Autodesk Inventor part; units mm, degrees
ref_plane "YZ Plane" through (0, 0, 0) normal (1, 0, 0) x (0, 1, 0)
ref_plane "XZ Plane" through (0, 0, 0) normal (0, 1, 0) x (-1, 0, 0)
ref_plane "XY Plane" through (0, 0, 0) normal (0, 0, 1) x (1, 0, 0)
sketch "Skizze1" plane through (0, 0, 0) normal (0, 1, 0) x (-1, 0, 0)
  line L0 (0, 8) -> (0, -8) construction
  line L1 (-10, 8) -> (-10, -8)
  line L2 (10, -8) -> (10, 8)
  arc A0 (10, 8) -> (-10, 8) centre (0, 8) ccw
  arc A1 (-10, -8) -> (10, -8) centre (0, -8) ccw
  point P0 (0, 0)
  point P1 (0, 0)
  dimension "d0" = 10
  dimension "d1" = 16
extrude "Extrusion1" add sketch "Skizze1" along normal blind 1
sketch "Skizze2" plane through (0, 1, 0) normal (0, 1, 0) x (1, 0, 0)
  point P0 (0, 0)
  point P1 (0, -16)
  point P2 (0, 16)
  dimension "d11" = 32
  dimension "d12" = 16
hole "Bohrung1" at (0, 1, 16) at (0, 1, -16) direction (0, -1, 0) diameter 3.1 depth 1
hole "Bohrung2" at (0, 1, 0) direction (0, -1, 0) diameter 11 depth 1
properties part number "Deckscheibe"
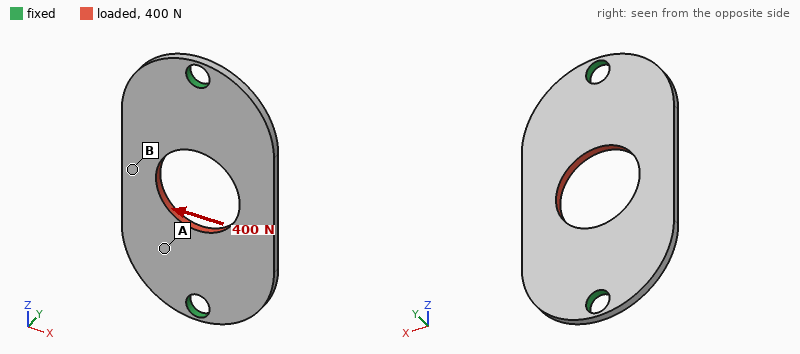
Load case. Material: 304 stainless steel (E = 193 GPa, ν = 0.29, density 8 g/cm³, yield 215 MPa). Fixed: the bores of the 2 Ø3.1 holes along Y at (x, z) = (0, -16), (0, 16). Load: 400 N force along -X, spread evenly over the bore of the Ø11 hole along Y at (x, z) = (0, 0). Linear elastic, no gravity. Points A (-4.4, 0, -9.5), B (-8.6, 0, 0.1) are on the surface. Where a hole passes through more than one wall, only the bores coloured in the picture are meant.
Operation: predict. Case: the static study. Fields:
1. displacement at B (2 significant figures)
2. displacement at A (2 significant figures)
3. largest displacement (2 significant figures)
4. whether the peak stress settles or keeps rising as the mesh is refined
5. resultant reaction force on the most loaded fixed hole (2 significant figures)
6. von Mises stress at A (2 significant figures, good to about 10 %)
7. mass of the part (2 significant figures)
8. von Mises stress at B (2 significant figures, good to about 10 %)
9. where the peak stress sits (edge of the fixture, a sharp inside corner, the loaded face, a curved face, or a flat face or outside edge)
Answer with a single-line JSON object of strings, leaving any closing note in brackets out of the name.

{"displacement at B": "3.8 µm", "displacement at A": "2.0 µm", "largest displacement": "4.0 µm", "whether the peak stress settles or keeps rising as the mesh is refined": "keeps rising", "resultant reaction force on the most loaded fixed hole": "200 N", "von Mises stress at A": "22 MPa", "mass of the part": "4.2 g", "von Mises stress at B": "36 MPa", "where the peak stress sits": "edge of the fixture"}
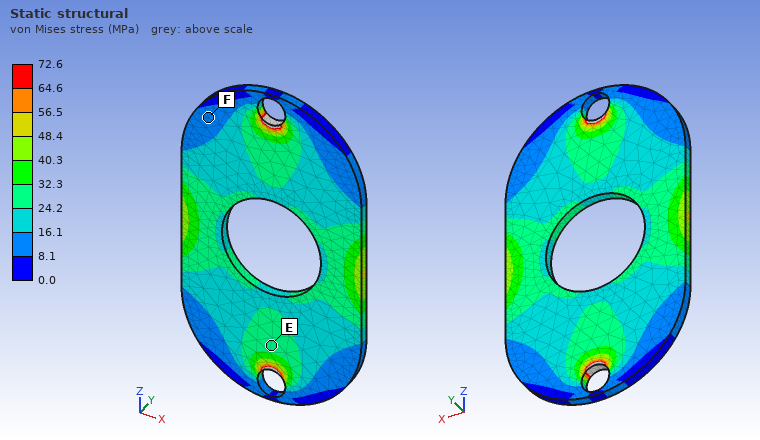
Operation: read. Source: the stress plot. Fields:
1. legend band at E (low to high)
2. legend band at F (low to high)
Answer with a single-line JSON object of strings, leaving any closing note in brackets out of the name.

{"legend band at E": "24.2 to 32.3 MPa", "legend band at F": "8.1 to 16.1 MPa"}
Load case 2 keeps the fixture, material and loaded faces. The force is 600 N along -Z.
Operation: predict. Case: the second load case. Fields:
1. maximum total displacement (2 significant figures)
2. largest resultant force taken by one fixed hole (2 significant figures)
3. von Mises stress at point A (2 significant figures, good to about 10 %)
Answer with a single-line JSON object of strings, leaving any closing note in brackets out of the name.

{"maximum total displacement": "2.3 µm", "largest resultant force taken by one fixed hole": "300 N", "von Mises stress at point A": "22 MPa"}
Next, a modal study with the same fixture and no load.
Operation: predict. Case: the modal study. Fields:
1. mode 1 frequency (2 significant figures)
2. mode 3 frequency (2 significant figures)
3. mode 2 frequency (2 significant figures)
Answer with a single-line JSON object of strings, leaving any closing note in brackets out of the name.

{"mode 1 frequency": "4500 Hz", "mode 3 frequency": "10 kHz", "mode 2 frequency": "4600 Hz"}
